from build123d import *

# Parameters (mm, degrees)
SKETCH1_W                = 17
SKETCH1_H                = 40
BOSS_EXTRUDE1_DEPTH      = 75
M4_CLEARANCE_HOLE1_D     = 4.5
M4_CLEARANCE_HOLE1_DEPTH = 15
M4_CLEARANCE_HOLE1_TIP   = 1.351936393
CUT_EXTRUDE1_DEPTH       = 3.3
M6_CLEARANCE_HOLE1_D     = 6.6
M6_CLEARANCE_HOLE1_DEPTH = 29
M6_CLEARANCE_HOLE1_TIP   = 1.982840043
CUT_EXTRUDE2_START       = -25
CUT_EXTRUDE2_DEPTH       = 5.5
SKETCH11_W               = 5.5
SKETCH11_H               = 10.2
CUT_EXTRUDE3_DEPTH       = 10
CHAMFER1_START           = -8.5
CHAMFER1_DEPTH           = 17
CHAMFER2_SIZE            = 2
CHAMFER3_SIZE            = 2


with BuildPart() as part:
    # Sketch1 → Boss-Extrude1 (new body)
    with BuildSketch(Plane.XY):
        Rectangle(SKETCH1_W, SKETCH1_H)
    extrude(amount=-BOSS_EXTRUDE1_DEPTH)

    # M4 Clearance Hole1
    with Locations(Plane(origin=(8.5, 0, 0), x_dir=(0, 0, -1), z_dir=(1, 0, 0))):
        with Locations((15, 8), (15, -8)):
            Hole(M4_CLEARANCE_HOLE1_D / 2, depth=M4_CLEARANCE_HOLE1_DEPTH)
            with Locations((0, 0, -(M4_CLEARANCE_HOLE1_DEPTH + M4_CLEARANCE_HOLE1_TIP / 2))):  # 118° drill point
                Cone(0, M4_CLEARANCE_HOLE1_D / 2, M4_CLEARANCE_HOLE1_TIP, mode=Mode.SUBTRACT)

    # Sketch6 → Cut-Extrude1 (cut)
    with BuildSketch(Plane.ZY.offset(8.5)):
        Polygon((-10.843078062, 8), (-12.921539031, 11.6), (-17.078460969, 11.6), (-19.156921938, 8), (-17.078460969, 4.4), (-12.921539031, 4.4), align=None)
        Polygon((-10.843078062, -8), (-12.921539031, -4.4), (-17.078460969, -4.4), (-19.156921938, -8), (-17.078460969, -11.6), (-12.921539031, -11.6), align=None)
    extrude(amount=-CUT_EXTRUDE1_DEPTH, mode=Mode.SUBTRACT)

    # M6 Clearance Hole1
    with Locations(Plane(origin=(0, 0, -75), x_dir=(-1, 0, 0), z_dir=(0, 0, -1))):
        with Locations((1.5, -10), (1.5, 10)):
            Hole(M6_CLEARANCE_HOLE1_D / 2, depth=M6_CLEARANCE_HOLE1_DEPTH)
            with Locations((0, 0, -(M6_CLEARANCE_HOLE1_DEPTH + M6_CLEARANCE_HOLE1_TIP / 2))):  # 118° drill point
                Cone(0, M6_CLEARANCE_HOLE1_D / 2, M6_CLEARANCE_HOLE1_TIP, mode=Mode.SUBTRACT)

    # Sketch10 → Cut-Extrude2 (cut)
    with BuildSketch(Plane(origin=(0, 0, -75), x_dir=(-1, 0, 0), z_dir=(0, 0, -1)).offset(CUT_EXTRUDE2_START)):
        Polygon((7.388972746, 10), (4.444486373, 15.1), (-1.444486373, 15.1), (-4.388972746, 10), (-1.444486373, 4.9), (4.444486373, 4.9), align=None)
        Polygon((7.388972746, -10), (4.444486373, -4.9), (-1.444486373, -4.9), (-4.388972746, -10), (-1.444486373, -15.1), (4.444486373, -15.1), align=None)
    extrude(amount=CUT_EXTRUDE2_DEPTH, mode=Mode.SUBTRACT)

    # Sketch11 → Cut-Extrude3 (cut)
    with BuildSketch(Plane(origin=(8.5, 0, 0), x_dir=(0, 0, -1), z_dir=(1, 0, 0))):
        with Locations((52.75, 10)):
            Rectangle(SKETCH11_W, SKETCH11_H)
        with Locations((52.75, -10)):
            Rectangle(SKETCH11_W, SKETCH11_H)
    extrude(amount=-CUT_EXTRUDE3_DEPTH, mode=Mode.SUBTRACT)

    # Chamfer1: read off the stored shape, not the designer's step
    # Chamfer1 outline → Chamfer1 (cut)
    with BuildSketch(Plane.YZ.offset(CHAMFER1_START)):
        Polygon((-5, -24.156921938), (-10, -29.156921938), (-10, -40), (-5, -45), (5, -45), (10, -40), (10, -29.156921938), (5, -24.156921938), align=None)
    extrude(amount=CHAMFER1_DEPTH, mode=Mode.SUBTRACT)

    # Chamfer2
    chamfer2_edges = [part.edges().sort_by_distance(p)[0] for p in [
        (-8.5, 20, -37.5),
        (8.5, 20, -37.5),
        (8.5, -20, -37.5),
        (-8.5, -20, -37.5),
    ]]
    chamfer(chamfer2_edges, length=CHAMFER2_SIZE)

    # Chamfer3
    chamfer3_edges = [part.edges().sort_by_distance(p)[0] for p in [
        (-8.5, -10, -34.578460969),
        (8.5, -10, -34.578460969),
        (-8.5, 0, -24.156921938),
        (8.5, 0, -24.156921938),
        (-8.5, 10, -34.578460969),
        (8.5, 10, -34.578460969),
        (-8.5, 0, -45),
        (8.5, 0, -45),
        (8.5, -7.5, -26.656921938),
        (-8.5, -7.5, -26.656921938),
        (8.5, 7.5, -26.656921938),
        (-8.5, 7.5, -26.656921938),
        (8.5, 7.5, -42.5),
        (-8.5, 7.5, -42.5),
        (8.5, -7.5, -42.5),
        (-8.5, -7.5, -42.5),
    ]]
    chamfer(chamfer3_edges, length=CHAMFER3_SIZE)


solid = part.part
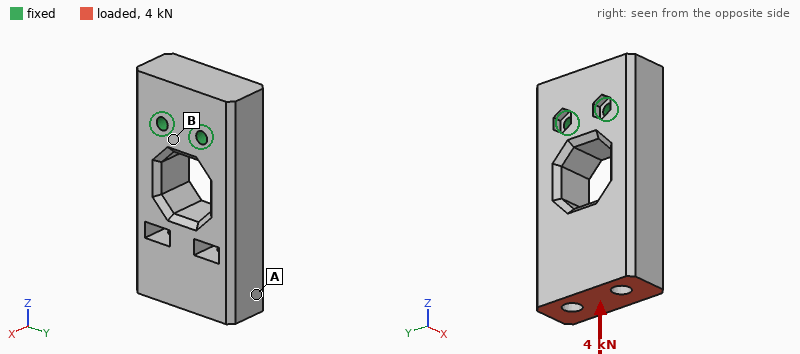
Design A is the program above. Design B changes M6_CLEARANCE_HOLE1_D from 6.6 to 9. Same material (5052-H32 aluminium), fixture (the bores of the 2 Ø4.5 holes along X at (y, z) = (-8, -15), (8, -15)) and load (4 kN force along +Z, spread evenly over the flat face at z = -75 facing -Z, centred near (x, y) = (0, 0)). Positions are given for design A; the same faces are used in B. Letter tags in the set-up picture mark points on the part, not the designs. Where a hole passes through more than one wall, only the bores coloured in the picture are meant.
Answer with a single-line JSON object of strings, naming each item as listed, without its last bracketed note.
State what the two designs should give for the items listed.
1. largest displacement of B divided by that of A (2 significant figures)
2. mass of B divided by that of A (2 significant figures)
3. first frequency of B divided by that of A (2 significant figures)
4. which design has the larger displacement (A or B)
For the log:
{"largest displacement of B divided by that of A": "1.1", "mass of B divided by that of A": "0.96", "first frequency of B divided by that of A": "1.0", "which design has the larger displacement": "B"}
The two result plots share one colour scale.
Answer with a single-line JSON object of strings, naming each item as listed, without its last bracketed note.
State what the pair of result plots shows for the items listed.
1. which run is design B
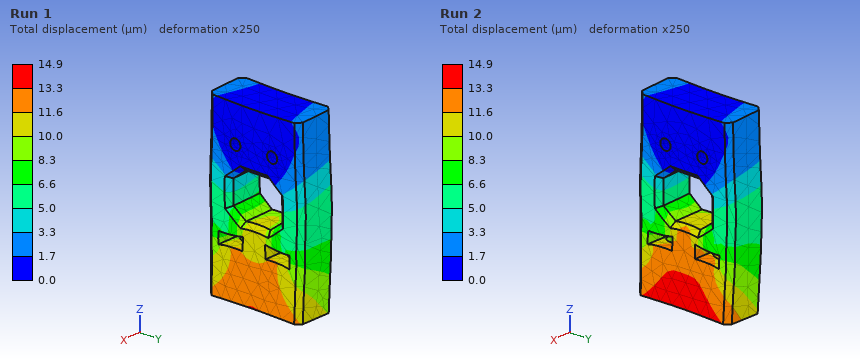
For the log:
{"which run is design B": "Run 2"}
